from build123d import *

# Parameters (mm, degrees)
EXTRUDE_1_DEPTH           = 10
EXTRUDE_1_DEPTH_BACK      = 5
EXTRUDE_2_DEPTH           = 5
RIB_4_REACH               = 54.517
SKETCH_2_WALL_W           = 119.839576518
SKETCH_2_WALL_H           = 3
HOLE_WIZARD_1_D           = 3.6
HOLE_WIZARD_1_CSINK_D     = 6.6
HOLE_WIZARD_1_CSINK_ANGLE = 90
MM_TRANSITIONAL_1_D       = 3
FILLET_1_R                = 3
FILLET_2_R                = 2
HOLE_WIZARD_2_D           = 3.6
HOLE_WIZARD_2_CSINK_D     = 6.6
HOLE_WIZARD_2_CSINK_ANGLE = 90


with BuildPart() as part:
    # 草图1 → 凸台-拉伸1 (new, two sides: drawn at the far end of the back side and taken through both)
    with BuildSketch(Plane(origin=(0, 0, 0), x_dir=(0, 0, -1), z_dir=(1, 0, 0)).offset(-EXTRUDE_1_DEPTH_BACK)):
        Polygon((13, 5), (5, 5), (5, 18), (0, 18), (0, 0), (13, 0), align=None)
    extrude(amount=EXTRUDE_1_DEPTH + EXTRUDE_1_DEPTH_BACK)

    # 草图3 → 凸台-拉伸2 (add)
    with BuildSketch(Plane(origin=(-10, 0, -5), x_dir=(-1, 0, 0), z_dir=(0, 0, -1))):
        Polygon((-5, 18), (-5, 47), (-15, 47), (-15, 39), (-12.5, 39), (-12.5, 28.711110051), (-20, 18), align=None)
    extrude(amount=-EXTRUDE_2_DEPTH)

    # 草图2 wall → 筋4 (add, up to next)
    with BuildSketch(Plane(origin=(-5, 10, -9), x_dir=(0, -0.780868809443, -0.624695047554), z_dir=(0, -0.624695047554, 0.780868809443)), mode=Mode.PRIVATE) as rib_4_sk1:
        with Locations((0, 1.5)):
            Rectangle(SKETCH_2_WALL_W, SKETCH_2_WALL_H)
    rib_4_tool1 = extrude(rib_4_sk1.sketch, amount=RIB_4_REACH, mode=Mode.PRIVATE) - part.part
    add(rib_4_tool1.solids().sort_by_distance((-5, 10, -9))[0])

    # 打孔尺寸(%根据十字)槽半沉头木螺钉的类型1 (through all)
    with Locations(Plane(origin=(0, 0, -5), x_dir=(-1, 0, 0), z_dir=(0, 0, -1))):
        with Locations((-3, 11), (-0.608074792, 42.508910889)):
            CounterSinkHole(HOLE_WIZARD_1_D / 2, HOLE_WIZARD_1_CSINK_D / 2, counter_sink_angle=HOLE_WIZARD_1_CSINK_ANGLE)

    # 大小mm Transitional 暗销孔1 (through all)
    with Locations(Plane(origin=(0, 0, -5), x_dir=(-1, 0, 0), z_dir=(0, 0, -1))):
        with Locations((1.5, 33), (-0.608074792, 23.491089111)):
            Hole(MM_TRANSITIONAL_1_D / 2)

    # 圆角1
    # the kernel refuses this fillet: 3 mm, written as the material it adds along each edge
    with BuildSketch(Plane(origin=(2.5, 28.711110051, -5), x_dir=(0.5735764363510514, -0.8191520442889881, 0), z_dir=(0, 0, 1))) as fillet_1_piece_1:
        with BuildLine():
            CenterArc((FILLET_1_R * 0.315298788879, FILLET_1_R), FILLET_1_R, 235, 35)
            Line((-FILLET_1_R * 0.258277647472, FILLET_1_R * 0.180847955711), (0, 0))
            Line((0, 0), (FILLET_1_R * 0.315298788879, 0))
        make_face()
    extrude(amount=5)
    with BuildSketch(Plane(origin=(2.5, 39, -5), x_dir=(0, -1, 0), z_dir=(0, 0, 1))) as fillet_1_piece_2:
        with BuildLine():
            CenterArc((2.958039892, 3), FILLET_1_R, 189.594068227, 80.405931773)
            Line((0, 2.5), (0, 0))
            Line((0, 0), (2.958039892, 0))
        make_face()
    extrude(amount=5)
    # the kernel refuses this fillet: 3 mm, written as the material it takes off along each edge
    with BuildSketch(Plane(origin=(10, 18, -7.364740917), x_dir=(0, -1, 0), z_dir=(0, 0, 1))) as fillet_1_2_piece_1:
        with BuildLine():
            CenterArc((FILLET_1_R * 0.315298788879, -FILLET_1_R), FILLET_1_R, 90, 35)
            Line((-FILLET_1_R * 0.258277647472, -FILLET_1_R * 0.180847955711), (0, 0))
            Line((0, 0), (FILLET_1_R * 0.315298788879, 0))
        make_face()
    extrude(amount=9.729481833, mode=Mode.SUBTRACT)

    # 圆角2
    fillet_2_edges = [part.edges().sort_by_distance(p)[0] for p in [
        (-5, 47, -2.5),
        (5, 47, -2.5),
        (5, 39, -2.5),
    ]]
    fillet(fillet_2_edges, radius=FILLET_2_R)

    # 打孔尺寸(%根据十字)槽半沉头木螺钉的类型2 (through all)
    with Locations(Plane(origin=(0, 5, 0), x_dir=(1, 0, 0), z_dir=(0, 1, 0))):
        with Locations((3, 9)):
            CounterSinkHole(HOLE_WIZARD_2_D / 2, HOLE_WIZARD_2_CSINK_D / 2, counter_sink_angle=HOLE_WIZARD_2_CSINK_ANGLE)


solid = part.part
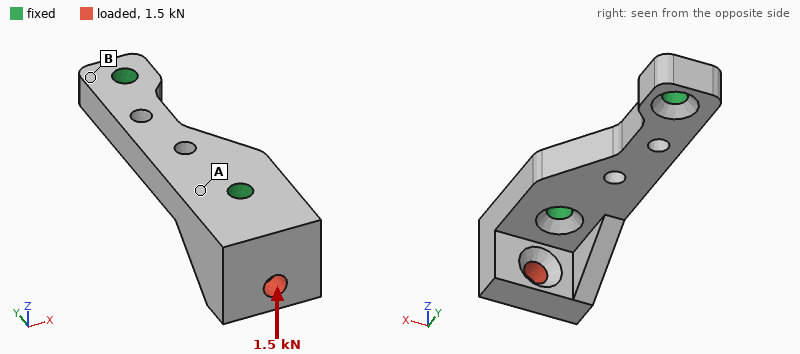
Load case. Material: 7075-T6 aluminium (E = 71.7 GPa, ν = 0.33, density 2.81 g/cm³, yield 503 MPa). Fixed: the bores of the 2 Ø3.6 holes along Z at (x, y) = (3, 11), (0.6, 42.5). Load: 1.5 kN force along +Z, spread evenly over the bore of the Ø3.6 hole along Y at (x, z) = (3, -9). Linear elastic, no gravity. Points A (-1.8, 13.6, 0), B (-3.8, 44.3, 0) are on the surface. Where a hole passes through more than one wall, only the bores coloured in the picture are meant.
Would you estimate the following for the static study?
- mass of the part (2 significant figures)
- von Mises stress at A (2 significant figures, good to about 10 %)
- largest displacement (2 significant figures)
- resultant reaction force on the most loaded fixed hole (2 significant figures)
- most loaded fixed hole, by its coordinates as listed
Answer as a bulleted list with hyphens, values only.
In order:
- 9.0 g
- 67 MPa
- 95 µm
- 1.6 kN
- (3, 11)
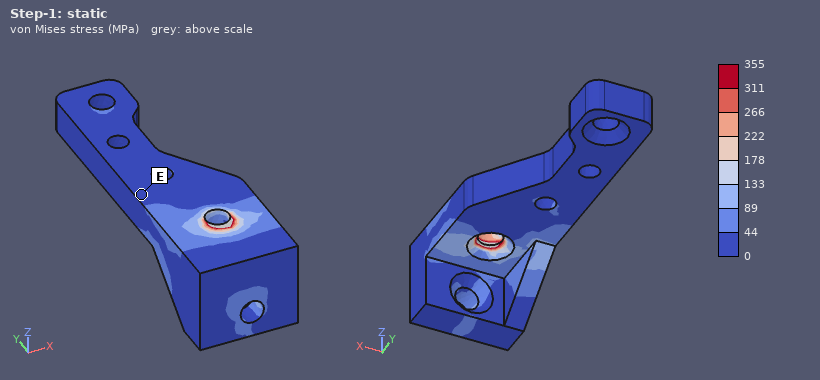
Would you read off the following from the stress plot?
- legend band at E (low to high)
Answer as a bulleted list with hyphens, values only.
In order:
- 0 to 44 MPa
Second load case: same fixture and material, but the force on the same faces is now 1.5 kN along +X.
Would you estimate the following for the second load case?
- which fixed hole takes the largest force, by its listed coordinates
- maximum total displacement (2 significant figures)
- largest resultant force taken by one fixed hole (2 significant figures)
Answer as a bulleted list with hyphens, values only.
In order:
- (3, 11)
- 0.10 mm
- 1.8 kN
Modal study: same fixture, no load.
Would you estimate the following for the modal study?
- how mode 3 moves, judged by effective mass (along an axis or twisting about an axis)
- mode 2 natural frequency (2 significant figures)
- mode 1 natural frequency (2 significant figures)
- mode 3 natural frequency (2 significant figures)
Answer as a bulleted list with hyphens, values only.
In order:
- along Z
- 16 kHz
- 13 kHz
- 23 kHz
